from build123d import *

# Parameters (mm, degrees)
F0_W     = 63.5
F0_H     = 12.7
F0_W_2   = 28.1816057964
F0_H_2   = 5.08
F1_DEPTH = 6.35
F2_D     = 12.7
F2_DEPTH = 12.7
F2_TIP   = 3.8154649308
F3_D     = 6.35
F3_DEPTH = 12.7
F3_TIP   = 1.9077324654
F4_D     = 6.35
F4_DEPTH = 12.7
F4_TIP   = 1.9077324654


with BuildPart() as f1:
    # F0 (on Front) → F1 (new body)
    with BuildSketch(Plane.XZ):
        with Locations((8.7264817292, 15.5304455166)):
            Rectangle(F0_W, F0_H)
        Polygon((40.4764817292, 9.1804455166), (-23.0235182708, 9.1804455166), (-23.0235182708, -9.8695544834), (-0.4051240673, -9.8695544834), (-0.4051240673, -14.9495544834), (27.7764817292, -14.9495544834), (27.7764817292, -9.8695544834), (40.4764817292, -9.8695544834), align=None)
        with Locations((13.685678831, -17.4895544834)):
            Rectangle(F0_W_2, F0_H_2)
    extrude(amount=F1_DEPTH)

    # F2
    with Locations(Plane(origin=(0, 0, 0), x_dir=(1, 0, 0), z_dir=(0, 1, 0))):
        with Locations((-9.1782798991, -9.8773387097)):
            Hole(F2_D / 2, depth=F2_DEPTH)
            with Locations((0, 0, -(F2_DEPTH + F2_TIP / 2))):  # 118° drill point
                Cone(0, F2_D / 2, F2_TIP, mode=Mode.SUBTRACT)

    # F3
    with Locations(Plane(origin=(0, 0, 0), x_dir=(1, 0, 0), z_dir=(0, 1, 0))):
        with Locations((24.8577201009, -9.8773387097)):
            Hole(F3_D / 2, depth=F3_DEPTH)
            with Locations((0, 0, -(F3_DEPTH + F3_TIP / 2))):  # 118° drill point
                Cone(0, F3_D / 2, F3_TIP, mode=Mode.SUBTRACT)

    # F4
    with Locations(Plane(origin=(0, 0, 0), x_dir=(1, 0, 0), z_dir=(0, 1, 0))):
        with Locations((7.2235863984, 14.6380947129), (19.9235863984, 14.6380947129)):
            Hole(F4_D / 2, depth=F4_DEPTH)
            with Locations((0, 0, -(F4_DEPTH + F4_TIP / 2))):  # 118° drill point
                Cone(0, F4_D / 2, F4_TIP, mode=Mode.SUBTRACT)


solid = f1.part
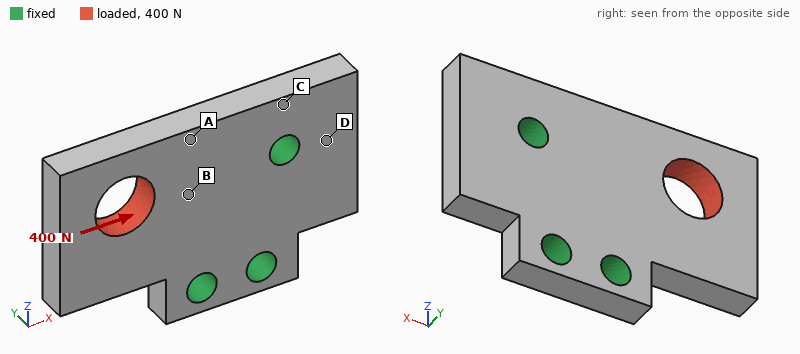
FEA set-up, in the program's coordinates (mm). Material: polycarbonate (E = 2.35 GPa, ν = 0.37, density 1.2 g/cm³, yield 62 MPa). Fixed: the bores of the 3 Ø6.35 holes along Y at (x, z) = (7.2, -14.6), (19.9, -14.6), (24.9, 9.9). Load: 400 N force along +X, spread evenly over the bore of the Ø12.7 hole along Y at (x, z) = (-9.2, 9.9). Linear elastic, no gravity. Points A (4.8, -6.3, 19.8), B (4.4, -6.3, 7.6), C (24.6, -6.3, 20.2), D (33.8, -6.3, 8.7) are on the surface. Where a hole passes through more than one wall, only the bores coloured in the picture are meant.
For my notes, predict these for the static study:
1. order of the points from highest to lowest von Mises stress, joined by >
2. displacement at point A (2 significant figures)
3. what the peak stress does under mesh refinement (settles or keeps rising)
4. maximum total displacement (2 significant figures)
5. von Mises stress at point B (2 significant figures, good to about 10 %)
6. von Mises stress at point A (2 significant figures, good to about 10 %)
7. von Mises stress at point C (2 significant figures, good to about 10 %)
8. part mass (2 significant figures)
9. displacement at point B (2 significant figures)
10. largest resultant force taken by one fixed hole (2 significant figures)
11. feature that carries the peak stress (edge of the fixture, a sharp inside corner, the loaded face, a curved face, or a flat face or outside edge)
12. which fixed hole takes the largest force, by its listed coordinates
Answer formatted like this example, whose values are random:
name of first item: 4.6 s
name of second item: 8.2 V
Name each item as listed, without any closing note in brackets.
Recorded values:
order of the points from highest to lowest von Mises stress, joined by >: A > B > C > D
displacement at point A: 37 µm
what the peak stress does under mesh refinement: keeps rising
maximum total displacement: 79 µm
von Mises stress at point B: 2.3 MPa
von Mises stress at point A: 3.4 MPa
von Mises stress at point C: 1.4 MPa
part mass: 16 g
displacement at point B: 22 µm
largest resultant force taken by one fixed hole: 340 N
feature that carries the peak stress: edge of the fixture
which fixed hole takes the largest force, by its listed coordinates: (24.9, 9.9)
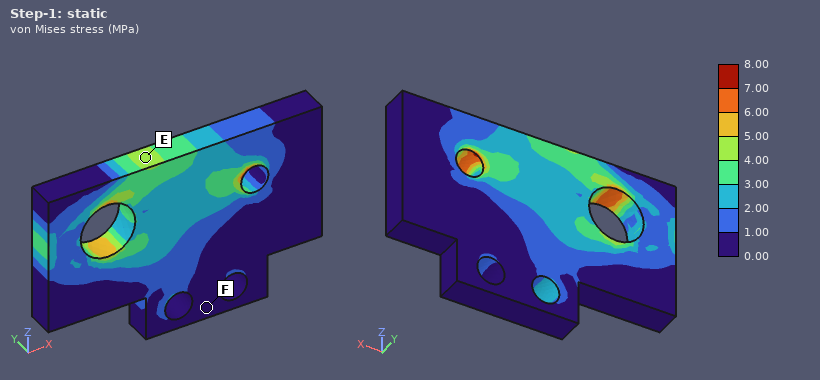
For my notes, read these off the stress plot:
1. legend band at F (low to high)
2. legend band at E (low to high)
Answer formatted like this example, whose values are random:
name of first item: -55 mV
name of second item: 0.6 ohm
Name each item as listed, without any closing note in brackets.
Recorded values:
legend band at F: 0.00 to 1.00 MPa
legend band at E: 4.00 to 5.00 MPa
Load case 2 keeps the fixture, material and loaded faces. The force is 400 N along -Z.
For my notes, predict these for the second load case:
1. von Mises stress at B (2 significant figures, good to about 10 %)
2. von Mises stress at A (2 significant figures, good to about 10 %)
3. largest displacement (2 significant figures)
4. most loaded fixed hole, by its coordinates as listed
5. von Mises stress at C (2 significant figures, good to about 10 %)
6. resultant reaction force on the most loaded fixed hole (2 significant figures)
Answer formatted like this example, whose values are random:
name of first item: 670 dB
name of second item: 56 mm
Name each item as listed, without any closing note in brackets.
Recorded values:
von Mises stress at B: 4.3 MPa
von Mises stress at A: 3.5 MPa
largest displacement: 0.16 mm
most loaded fixed hole, by its coordinates as listed: (7.2, -14.6)
von Mises stress at C: 1.7 MPa
resultant reaction force on the most loaded fixed hole: 400 N
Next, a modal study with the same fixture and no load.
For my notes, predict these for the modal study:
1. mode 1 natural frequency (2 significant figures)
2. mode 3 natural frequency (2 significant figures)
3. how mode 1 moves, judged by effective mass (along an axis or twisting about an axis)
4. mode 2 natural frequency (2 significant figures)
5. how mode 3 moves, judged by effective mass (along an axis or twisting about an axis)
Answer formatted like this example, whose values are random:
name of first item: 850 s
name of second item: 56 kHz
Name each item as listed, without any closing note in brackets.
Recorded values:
mode 1 natural frequency: 1000 Hz
mode 3 natural frequency: 3700 Hz
how mode 1 moves, judged by effective mass: along Y
mode 2 natural frequency: 2400 Hz
how mode 3 moves, judged by effective mass: along Z
